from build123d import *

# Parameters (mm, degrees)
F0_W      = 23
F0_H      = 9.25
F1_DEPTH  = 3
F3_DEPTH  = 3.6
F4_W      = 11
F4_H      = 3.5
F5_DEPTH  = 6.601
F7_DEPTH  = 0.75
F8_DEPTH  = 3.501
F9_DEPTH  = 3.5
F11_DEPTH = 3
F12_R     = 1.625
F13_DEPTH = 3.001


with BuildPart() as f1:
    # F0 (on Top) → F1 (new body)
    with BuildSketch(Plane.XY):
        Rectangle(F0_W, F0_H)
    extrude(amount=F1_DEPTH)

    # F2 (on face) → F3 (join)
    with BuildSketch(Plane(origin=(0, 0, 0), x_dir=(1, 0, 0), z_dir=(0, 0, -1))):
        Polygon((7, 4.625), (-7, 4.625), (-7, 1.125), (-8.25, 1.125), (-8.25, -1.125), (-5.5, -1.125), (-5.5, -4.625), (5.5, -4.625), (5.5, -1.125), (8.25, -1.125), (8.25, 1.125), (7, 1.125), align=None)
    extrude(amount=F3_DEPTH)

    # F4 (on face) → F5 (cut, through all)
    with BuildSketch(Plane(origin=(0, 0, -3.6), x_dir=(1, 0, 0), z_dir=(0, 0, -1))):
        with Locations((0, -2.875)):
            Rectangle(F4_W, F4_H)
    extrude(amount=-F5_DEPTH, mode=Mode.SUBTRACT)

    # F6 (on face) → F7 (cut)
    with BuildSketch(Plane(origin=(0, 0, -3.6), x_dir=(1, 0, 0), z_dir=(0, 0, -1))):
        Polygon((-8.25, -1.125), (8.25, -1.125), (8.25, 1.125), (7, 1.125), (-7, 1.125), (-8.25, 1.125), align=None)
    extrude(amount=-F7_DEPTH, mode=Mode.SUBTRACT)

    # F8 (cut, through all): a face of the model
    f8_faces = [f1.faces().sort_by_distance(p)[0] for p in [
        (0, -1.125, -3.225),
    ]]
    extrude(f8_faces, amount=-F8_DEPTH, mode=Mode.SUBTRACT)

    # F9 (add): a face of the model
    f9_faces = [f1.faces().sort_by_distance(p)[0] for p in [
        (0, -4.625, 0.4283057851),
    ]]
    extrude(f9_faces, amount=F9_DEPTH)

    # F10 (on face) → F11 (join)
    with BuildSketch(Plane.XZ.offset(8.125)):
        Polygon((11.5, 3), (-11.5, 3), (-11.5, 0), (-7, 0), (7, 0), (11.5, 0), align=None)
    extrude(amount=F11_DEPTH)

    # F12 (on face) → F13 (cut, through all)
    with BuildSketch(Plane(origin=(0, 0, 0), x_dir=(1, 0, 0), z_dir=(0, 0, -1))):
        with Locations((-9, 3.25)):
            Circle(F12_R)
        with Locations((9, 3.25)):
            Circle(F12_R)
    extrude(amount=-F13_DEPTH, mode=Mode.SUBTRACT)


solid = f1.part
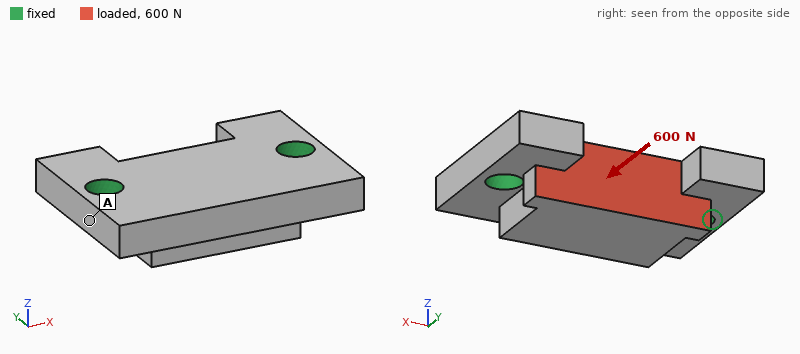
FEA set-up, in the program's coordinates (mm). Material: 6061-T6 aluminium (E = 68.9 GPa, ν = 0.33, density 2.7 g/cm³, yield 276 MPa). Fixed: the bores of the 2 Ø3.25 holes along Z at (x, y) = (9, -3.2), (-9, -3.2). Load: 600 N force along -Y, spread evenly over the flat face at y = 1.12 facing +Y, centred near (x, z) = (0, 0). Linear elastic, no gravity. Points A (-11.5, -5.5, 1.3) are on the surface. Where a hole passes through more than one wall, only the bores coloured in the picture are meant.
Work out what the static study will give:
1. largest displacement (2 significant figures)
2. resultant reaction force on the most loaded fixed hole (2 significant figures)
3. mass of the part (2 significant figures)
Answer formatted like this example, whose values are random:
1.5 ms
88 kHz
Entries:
4.9 µm
300 N
3.5 g
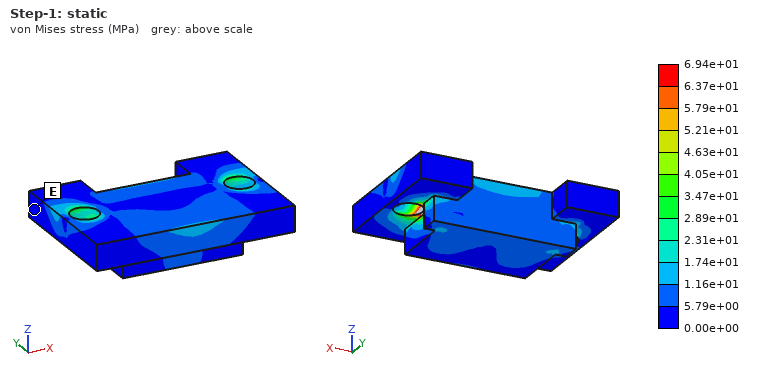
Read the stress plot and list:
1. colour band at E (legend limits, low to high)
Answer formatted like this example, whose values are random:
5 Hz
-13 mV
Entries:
0.00e+00 to 5.79e+00 MPa
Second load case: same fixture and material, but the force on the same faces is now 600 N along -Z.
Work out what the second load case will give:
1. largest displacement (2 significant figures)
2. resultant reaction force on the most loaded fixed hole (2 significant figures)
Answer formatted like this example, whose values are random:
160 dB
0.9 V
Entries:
13 µm
340 N
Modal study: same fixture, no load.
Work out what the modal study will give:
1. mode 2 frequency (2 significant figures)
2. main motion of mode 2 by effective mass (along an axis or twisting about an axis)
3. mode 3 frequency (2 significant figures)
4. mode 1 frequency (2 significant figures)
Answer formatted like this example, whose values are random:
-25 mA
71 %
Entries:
47 kHz
along Z
57 kHz
31 kHz
